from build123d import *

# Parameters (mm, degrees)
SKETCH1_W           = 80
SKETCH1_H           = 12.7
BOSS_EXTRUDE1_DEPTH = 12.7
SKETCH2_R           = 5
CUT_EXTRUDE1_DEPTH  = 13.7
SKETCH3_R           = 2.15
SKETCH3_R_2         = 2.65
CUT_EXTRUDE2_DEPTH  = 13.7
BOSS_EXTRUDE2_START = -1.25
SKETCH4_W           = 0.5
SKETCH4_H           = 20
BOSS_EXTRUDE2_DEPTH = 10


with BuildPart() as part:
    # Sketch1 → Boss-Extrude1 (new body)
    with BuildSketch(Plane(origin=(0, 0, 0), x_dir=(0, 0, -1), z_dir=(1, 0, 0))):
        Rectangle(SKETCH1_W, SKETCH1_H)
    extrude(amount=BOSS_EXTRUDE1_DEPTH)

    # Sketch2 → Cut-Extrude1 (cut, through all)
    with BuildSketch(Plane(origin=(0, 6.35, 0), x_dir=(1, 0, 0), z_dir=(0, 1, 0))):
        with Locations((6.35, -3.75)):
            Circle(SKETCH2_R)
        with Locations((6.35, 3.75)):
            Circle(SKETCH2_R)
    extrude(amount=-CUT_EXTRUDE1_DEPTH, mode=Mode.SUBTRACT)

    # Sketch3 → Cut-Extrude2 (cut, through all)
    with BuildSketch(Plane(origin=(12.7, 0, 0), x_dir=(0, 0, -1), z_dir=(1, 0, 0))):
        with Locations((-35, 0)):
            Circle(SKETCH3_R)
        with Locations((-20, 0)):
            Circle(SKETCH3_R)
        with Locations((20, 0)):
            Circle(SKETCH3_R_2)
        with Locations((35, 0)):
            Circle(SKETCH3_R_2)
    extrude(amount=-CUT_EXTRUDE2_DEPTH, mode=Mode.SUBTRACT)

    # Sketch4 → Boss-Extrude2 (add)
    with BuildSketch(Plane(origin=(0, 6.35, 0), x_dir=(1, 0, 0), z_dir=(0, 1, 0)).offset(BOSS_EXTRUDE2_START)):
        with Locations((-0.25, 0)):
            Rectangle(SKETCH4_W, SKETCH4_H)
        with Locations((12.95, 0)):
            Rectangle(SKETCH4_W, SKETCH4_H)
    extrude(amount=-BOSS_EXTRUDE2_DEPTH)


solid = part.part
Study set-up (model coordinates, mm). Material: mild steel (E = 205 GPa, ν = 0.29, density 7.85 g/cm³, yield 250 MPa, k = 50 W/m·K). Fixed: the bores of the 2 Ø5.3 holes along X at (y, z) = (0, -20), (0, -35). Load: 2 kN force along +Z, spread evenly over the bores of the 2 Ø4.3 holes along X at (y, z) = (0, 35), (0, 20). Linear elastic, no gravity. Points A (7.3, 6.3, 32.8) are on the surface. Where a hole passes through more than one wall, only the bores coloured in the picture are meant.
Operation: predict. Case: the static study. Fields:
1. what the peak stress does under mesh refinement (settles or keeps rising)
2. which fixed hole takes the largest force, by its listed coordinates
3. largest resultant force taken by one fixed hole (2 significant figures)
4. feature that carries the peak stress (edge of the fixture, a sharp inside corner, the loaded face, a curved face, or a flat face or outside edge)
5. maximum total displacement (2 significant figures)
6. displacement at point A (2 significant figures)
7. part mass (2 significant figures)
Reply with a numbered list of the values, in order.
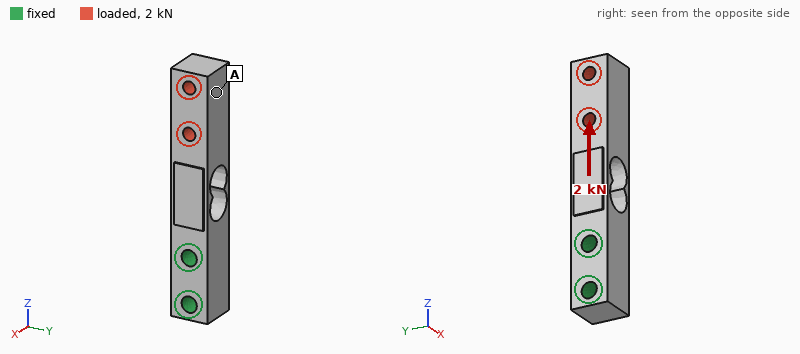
1. keeps rising
2. (0, -20)
3. 1.9 kN
4. a sharp inside corner
5. 6.7 µm
6. 6.3 µm
7. 81 g
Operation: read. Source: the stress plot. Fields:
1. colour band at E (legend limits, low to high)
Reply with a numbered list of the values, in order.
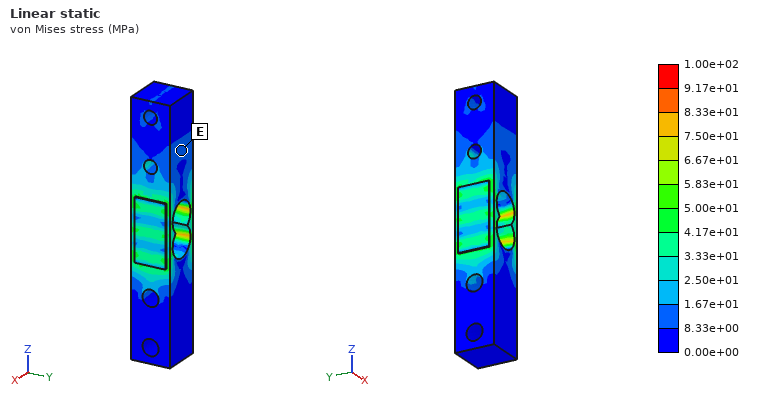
1. 8.33e+00 to 1.67e+01 MPa
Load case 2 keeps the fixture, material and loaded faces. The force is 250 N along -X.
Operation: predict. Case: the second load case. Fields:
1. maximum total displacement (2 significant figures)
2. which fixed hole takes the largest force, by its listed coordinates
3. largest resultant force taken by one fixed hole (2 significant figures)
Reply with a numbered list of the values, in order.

1. 54 µm
2. (0, -20)
3. 310 N
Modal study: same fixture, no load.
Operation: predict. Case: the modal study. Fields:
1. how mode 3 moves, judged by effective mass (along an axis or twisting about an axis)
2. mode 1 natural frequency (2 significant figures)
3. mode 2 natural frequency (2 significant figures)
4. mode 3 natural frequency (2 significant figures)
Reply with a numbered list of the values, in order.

1. twisting about Z
2. 2000 Hz
3. 2000 Hz
4. 8000 Hz
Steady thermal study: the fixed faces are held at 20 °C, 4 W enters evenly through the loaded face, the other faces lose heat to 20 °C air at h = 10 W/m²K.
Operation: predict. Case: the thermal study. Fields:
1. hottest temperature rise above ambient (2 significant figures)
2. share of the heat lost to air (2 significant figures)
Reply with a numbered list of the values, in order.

1. 35 K
2. 18 %
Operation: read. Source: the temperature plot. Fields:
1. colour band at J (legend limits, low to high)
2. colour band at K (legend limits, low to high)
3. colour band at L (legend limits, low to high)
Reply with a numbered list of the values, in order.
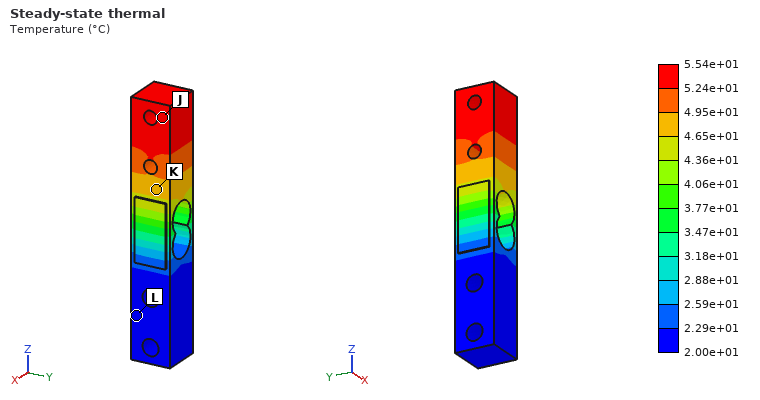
1. 5.24e+01 to 5.54e+01 °C
2. 4.65e+01 to 4.95e+01 °C
3. 2.00e+01 to 2.29e+01 °C
